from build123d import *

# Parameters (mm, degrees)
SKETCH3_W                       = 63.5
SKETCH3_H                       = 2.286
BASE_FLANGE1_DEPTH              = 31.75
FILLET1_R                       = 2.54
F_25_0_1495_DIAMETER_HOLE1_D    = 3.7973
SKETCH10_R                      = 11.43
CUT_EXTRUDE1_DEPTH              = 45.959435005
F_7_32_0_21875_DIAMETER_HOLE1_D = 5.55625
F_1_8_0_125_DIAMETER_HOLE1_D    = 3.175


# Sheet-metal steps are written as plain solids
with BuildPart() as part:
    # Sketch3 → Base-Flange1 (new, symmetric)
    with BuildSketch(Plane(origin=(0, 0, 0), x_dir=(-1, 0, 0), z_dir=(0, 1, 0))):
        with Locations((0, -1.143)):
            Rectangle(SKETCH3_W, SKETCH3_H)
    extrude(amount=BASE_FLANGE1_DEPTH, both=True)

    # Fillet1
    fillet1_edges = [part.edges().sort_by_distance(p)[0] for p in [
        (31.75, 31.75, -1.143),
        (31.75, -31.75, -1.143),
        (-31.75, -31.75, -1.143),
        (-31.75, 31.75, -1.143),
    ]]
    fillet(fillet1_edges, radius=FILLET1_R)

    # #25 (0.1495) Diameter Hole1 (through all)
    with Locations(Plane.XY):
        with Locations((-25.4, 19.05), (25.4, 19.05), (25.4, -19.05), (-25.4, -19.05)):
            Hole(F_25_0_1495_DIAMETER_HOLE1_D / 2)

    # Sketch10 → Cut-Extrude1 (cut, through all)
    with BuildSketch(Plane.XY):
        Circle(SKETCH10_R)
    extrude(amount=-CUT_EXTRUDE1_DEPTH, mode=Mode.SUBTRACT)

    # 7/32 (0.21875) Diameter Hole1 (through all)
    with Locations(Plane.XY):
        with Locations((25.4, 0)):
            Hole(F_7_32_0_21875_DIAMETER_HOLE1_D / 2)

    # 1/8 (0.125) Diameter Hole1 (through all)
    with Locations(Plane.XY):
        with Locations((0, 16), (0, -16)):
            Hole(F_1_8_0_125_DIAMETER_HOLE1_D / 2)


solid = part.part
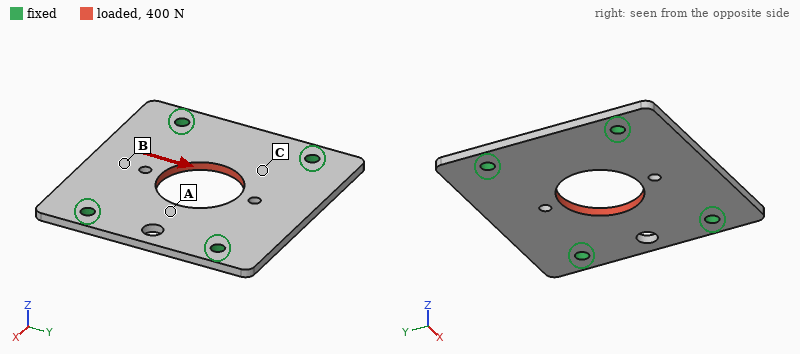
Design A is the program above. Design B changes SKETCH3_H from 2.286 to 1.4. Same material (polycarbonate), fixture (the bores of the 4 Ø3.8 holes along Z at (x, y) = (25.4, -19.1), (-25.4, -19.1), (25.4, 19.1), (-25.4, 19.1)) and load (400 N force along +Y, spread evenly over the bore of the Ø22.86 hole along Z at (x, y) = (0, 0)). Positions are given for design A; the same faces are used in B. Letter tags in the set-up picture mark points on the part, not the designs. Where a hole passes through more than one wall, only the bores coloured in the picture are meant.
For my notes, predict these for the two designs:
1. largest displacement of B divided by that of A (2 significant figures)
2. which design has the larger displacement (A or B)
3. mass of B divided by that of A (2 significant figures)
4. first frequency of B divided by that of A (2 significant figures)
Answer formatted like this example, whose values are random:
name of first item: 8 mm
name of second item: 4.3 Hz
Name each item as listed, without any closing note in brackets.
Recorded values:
largest displacement of B divided by that of A: 1.6
which design has the larger displacement: B
mass of B divided by that of A: 0.61
first frequency of B divided by that of A: 0.64
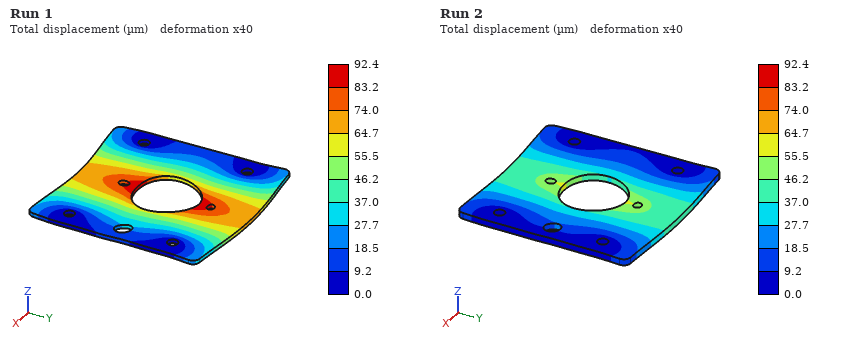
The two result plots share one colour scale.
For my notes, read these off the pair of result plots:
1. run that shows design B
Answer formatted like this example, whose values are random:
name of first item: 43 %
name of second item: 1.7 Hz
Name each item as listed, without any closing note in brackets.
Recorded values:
run that shows design B: Run 1
